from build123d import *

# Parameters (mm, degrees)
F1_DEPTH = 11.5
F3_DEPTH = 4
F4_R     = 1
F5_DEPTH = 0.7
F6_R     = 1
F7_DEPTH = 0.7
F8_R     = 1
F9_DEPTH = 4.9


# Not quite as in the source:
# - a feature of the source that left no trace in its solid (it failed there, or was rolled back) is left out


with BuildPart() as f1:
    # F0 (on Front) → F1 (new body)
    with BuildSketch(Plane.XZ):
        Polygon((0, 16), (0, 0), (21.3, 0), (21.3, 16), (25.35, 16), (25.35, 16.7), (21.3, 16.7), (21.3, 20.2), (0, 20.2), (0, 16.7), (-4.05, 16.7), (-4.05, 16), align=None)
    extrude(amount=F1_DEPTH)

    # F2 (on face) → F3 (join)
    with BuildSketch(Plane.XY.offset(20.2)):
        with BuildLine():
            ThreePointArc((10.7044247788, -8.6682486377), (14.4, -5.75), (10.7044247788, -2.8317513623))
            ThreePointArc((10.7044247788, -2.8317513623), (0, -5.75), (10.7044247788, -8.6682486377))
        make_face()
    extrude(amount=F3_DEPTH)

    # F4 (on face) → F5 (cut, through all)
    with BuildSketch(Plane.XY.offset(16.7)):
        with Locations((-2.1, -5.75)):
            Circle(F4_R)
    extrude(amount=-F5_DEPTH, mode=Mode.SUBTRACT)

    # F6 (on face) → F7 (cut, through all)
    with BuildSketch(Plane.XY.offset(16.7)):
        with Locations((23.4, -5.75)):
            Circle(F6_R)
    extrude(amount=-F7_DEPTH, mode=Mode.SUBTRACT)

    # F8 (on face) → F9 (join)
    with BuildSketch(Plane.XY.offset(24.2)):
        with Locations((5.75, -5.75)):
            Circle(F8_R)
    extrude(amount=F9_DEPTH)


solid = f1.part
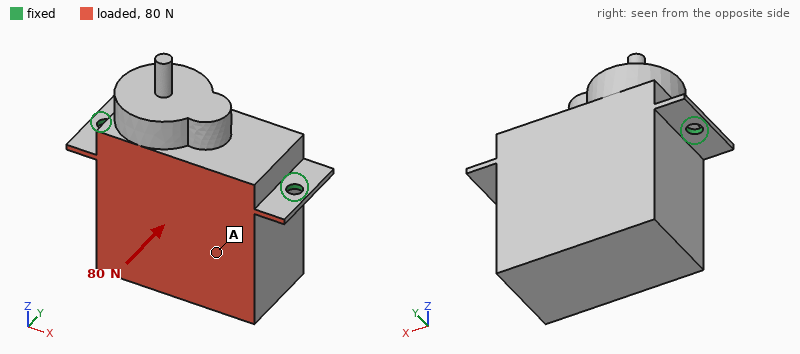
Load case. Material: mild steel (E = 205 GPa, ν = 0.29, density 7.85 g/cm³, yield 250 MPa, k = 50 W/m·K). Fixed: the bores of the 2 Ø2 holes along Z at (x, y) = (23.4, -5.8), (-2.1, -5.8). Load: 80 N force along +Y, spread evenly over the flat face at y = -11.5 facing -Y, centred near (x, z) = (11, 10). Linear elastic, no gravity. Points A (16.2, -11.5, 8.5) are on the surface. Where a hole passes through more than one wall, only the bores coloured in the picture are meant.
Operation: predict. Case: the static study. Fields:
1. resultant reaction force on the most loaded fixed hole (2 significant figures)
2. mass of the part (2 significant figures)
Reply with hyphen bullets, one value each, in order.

- 40 N
- 43 g
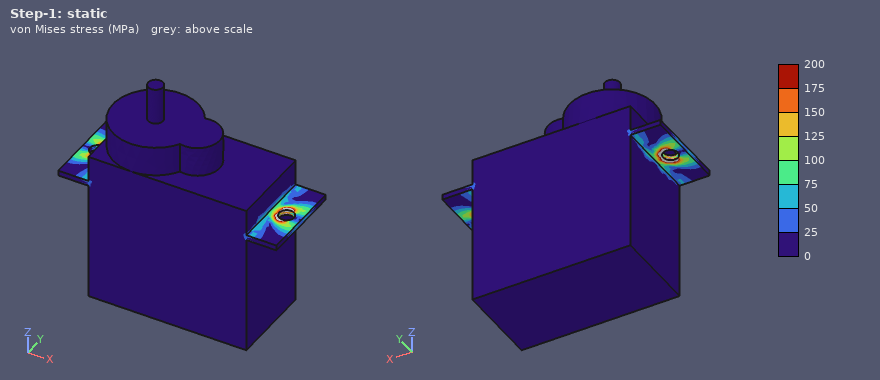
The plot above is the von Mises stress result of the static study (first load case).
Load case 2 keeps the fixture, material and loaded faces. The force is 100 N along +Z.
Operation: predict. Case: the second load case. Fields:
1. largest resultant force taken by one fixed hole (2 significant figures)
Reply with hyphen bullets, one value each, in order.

- 50 N
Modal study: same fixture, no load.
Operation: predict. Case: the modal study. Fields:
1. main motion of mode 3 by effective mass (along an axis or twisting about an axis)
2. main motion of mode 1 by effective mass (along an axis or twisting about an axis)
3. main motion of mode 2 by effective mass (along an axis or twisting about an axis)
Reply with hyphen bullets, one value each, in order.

- along X
- along Y
- along Z
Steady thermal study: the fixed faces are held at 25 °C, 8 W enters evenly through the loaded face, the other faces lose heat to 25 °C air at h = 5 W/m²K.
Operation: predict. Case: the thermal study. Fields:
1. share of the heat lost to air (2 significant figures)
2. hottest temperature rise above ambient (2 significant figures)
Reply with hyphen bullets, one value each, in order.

- 3.8 %
- 41 K
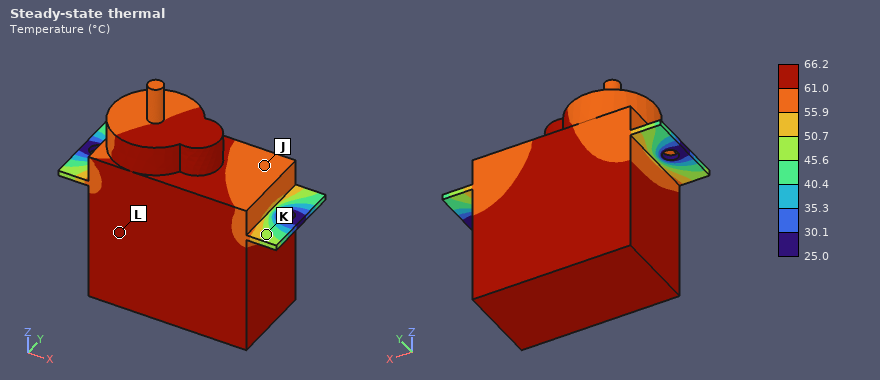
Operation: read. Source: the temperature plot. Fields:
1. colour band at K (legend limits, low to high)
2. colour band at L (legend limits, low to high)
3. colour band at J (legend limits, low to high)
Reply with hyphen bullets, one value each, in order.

- 45.6 to 50.7 °C
- 61.0 to 66.2 °C
- 55.9 to 61.0 °C
